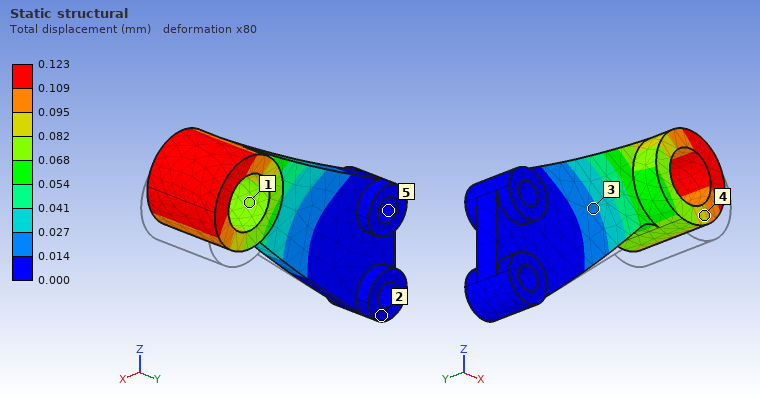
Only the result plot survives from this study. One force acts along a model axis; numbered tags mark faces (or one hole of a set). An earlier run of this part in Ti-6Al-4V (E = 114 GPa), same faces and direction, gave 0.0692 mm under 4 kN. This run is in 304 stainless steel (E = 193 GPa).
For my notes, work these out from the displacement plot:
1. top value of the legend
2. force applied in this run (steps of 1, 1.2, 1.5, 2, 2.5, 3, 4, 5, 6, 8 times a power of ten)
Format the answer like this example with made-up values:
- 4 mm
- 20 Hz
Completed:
- 0.123 mm
- 12 kN
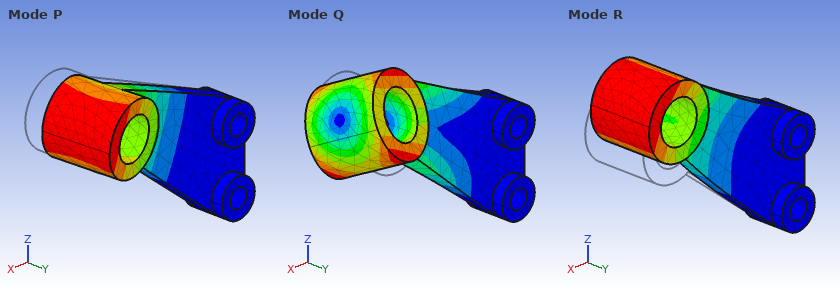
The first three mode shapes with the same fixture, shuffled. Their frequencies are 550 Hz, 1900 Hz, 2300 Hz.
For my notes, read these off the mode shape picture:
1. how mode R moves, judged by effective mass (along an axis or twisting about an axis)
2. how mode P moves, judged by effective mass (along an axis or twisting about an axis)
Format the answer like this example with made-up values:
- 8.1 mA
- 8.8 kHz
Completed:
- along Z
- along Y
